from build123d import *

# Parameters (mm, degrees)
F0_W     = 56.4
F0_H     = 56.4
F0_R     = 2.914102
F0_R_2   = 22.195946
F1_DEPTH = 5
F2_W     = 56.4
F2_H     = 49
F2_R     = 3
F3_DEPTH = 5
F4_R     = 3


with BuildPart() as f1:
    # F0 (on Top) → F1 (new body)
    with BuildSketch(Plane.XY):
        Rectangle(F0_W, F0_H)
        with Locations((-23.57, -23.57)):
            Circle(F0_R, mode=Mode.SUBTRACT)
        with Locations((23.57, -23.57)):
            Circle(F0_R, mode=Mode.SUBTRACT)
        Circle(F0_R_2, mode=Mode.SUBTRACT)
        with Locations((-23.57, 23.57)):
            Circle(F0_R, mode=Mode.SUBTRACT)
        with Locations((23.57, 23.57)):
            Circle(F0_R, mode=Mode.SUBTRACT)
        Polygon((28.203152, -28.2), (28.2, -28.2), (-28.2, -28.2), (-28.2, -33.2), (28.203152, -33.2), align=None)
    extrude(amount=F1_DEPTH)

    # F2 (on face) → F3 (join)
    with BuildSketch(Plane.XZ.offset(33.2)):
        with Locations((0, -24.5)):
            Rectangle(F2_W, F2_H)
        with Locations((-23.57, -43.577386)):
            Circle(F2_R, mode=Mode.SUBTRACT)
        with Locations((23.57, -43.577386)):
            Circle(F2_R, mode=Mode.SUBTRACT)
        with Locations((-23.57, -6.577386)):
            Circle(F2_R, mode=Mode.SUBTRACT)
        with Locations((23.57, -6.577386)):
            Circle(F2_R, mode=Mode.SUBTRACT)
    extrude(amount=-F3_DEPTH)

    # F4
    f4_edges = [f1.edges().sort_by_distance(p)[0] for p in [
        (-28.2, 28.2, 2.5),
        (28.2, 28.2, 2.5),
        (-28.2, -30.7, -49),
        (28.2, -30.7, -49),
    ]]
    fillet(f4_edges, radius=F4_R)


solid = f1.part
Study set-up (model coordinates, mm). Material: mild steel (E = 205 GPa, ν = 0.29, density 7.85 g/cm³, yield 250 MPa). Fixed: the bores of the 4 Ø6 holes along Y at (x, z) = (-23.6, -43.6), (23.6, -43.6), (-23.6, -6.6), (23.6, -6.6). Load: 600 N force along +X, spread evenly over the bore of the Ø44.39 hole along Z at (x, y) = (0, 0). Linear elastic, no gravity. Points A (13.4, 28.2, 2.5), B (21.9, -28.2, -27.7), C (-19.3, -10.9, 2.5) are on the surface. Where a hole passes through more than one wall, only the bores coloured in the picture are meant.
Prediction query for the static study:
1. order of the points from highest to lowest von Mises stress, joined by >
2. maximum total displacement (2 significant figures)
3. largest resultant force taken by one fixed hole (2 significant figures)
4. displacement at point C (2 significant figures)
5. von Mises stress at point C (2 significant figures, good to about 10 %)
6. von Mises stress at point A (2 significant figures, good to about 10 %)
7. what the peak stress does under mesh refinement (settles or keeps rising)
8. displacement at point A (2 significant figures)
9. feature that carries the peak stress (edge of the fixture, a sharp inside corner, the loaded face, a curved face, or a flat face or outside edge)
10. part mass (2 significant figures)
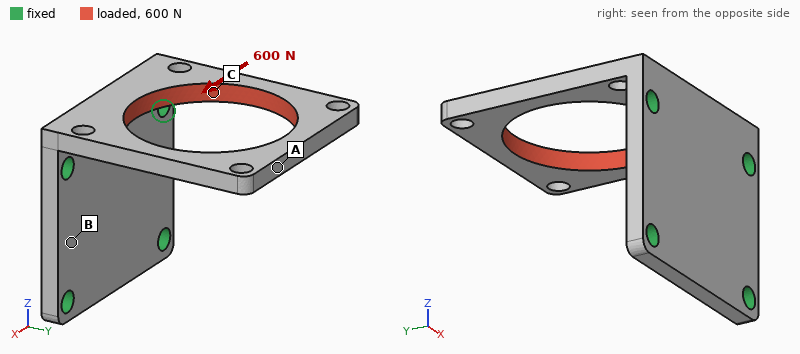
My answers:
C > A > B
28 µm
480 N
6.1 µm
35 MPa
15 MPa
keeps rising
27 µm
edge of the fixture
170 g
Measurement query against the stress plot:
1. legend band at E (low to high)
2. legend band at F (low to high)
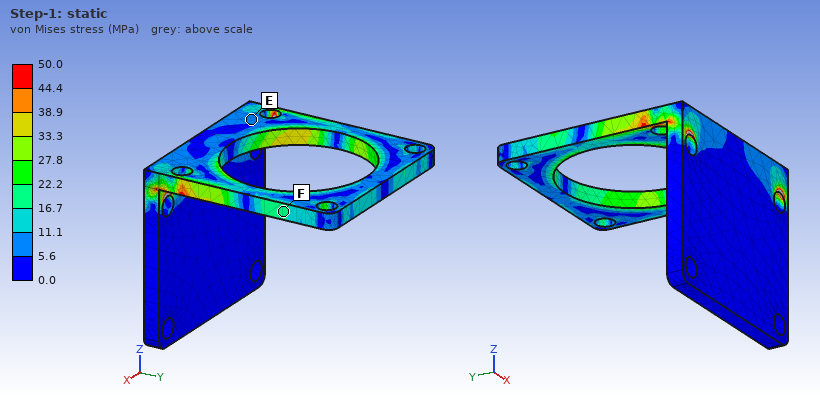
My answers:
5.6 to 11.1 MPa
16.7 to 22.2 MPa
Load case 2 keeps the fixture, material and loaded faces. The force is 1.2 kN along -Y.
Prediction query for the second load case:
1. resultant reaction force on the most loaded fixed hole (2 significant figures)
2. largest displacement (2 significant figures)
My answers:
620 N
28 µm
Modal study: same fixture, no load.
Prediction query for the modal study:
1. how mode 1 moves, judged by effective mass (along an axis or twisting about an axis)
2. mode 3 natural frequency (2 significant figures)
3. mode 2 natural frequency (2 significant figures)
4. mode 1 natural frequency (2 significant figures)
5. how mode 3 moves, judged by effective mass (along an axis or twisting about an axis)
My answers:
along Z
3300 Hz
2100 Hz
870 Hz
along X
